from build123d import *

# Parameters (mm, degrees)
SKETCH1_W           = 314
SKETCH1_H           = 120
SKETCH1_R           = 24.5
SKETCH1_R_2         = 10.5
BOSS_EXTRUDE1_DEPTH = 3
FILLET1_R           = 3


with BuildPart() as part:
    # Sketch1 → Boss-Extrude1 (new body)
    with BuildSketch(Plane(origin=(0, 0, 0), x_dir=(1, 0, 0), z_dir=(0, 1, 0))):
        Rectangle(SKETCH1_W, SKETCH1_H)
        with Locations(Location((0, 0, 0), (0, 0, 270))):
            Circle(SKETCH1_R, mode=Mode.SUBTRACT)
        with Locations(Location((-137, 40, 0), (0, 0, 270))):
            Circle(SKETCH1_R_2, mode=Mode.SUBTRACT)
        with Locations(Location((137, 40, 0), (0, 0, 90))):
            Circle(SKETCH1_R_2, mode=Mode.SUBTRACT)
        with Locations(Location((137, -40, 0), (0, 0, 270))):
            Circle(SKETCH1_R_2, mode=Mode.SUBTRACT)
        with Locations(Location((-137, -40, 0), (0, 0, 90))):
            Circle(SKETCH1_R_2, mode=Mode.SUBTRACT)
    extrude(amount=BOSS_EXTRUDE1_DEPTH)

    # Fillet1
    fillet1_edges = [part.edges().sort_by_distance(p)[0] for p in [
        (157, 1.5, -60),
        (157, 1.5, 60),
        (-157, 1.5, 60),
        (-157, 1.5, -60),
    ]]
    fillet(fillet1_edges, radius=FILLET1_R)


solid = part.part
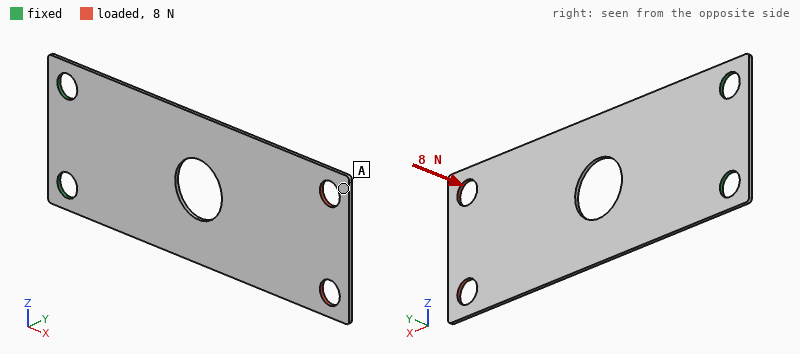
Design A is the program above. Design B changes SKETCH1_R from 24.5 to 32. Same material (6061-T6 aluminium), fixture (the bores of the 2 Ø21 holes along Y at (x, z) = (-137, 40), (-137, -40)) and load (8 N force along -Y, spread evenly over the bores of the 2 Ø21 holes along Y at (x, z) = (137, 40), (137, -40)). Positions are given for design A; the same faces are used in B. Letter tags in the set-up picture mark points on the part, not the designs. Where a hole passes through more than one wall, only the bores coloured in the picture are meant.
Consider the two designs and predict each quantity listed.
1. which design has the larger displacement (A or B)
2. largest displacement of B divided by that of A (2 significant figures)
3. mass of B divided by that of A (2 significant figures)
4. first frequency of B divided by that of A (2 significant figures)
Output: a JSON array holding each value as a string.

["B", "1.1", "0.96", "0.97"]
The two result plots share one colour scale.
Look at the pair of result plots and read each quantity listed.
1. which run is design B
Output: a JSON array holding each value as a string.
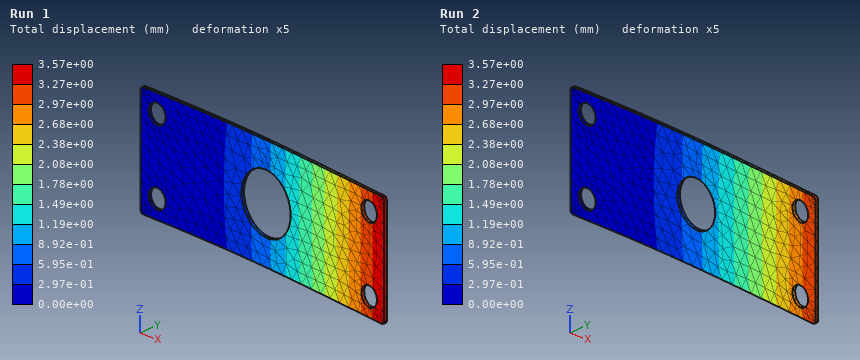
["Run 1"]
